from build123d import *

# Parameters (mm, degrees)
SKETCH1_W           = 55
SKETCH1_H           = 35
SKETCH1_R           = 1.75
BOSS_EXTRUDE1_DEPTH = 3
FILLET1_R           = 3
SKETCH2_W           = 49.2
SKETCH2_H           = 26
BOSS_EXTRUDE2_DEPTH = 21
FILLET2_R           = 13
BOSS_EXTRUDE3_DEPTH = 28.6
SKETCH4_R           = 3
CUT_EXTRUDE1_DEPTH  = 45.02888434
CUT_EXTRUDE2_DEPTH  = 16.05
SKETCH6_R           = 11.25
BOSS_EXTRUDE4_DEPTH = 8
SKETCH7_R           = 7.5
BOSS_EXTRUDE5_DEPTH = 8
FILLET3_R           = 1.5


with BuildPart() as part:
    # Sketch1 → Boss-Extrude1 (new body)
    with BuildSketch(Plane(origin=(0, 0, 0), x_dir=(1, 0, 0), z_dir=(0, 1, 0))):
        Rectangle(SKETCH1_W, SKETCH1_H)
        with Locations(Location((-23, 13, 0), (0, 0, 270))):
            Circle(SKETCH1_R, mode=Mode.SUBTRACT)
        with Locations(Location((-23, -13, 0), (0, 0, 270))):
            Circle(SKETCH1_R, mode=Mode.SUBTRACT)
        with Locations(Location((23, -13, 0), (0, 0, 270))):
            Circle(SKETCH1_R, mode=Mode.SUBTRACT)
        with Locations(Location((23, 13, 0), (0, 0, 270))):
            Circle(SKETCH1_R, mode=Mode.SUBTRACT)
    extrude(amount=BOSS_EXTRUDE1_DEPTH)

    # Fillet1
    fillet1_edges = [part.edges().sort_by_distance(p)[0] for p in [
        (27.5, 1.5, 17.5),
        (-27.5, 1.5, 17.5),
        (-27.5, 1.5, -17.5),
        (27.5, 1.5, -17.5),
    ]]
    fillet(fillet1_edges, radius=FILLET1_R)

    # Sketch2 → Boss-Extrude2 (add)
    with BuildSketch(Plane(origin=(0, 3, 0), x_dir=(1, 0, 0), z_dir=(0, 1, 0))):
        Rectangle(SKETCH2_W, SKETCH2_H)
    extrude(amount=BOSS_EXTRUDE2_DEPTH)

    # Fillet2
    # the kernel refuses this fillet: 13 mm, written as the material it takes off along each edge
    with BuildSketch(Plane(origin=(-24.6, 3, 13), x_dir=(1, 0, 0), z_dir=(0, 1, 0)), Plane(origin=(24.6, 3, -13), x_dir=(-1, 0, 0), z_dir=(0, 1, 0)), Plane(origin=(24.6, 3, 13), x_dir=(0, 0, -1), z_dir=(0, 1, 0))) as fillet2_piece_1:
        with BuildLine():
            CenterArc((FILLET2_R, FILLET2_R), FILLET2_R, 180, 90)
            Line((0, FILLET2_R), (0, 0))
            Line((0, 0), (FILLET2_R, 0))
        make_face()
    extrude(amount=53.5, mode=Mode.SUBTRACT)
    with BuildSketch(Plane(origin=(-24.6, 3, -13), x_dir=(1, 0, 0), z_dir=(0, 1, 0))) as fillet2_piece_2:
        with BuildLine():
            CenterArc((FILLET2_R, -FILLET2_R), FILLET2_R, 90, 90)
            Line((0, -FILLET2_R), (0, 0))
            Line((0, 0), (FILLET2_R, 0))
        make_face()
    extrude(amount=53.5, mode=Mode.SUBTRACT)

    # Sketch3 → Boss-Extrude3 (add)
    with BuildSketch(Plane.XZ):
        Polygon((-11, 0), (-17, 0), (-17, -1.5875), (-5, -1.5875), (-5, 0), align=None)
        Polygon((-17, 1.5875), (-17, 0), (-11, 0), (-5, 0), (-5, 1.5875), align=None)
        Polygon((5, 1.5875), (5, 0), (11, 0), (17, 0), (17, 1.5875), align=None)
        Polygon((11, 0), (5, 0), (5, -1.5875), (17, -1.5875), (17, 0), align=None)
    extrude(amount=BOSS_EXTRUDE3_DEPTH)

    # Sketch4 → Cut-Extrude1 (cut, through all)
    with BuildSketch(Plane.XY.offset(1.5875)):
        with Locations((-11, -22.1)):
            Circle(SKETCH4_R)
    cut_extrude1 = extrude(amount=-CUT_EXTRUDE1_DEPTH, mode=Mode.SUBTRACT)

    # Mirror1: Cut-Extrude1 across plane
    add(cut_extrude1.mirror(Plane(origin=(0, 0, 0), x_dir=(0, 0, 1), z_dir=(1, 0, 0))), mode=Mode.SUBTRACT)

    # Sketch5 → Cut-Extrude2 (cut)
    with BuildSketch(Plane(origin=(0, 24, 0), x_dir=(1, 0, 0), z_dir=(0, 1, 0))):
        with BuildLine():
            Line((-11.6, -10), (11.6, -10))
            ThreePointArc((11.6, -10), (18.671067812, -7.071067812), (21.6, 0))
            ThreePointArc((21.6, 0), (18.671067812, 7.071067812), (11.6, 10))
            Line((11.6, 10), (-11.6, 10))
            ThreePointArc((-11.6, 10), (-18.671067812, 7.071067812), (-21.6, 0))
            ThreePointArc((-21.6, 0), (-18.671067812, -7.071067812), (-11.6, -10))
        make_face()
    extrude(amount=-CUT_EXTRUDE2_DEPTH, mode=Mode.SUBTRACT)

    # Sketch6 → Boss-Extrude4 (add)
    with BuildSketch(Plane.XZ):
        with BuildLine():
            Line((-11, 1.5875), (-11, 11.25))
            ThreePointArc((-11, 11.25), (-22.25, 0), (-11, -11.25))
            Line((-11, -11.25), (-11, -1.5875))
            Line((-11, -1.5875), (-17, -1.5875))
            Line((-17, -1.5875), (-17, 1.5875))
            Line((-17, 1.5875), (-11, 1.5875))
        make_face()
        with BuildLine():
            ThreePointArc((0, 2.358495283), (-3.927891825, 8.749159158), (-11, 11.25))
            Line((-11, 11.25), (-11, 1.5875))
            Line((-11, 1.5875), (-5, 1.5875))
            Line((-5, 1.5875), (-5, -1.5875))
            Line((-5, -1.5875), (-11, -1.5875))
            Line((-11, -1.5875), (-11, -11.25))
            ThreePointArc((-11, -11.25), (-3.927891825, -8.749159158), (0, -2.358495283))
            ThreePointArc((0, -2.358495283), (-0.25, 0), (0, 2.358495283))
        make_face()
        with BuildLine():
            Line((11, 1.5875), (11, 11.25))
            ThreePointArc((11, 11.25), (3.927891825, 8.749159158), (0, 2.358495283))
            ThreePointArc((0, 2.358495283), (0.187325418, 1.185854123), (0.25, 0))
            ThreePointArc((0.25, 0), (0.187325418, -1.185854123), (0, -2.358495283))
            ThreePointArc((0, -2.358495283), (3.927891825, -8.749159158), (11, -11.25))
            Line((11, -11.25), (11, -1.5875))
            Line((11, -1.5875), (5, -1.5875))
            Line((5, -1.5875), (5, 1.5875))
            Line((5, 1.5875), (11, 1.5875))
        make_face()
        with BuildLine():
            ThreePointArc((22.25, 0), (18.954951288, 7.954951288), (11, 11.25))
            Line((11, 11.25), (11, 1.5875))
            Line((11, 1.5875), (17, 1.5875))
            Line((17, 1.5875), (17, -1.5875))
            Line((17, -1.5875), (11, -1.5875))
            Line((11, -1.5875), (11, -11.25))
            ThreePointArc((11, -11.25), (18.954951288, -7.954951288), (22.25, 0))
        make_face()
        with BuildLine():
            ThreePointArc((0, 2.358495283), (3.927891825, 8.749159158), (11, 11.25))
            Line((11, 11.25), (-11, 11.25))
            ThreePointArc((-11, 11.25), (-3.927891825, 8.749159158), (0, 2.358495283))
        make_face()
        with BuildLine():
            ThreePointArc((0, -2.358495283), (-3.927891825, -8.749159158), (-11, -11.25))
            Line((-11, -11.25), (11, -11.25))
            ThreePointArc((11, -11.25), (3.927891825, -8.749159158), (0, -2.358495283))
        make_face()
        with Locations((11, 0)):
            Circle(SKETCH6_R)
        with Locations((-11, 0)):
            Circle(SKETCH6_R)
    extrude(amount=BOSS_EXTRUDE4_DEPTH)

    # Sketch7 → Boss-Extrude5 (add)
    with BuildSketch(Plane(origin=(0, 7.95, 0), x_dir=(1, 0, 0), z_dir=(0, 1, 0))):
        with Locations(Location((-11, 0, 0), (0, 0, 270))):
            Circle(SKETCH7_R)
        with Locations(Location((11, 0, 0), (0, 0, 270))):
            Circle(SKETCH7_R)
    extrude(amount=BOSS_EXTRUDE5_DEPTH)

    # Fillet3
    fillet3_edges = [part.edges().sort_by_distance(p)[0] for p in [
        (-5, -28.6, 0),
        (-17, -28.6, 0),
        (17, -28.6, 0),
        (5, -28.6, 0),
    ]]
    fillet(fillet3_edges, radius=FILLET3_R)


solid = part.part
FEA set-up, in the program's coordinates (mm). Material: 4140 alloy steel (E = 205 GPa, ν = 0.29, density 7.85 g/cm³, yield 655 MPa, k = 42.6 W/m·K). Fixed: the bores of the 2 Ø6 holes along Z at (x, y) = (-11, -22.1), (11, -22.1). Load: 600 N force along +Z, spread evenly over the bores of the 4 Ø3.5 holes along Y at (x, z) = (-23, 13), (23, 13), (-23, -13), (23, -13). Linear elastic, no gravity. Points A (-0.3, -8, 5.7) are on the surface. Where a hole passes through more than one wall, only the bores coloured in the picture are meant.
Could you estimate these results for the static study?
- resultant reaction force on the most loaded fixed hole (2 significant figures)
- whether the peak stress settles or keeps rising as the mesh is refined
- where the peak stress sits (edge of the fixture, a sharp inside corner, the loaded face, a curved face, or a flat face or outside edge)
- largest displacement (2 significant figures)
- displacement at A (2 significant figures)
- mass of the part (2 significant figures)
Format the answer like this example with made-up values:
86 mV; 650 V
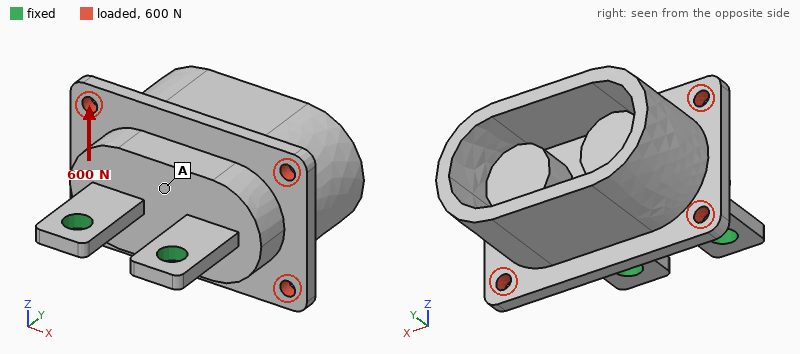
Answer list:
300 N; keeps rising; edge of the fixture; 0.35 mm; 0.074 mm; 220 g
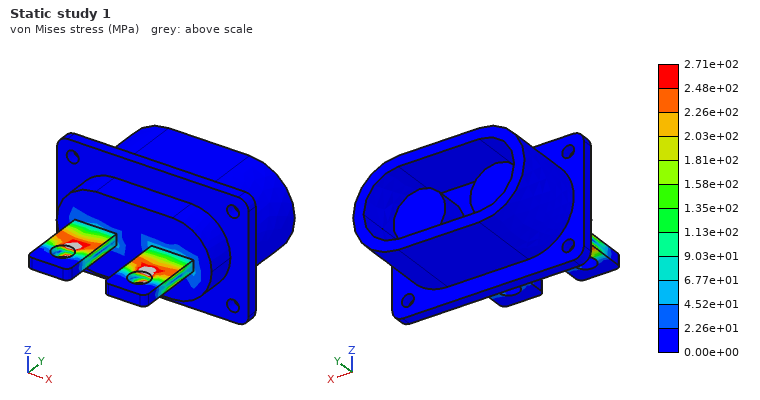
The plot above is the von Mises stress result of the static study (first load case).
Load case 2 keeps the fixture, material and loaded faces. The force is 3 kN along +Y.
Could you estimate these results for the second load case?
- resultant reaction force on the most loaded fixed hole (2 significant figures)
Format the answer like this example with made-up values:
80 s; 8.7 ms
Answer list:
1.5 kN
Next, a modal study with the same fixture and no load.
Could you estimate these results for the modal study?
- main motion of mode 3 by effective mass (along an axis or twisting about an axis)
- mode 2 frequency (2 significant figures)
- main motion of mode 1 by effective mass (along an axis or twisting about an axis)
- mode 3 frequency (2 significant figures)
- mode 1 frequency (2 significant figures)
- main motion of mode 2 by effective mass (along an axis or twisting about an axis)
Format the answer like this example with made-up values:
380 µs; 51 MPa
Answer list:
along X; 2100 Hz; along Z; 3800 Hz; 510 Hz; twisting about Y
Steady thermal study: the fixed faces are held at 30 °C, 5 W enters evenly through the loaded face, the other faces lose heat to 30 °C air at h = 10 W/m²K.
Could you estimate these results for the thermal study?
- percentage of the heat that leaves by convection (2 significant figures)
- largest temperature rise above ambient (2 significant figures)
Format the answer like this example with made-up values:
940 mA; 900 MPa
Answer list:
33 %; 22 K
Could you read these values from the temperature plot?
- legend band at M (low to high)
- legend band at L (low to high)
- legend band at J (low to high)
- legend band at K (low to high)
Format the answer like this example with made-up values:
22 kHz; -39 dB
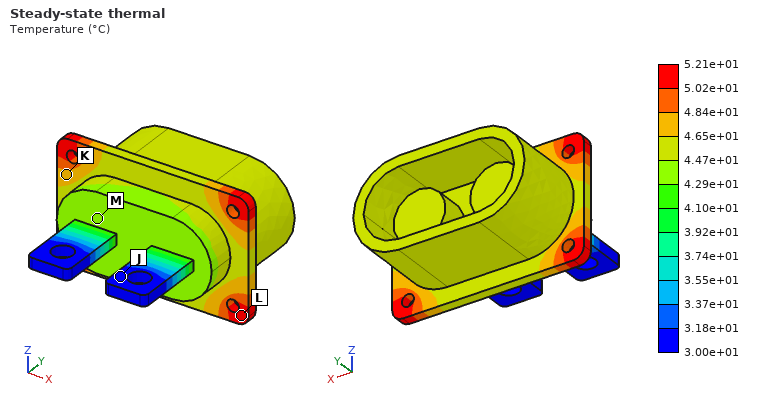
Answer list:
4.29e+01 to 4.47e+01 °C; 5.02e+01 to 5.21e+01 °C; 3.00e+01 to 3.18e+01 °C; 4.65e+01 to 4.84e+01 °C
